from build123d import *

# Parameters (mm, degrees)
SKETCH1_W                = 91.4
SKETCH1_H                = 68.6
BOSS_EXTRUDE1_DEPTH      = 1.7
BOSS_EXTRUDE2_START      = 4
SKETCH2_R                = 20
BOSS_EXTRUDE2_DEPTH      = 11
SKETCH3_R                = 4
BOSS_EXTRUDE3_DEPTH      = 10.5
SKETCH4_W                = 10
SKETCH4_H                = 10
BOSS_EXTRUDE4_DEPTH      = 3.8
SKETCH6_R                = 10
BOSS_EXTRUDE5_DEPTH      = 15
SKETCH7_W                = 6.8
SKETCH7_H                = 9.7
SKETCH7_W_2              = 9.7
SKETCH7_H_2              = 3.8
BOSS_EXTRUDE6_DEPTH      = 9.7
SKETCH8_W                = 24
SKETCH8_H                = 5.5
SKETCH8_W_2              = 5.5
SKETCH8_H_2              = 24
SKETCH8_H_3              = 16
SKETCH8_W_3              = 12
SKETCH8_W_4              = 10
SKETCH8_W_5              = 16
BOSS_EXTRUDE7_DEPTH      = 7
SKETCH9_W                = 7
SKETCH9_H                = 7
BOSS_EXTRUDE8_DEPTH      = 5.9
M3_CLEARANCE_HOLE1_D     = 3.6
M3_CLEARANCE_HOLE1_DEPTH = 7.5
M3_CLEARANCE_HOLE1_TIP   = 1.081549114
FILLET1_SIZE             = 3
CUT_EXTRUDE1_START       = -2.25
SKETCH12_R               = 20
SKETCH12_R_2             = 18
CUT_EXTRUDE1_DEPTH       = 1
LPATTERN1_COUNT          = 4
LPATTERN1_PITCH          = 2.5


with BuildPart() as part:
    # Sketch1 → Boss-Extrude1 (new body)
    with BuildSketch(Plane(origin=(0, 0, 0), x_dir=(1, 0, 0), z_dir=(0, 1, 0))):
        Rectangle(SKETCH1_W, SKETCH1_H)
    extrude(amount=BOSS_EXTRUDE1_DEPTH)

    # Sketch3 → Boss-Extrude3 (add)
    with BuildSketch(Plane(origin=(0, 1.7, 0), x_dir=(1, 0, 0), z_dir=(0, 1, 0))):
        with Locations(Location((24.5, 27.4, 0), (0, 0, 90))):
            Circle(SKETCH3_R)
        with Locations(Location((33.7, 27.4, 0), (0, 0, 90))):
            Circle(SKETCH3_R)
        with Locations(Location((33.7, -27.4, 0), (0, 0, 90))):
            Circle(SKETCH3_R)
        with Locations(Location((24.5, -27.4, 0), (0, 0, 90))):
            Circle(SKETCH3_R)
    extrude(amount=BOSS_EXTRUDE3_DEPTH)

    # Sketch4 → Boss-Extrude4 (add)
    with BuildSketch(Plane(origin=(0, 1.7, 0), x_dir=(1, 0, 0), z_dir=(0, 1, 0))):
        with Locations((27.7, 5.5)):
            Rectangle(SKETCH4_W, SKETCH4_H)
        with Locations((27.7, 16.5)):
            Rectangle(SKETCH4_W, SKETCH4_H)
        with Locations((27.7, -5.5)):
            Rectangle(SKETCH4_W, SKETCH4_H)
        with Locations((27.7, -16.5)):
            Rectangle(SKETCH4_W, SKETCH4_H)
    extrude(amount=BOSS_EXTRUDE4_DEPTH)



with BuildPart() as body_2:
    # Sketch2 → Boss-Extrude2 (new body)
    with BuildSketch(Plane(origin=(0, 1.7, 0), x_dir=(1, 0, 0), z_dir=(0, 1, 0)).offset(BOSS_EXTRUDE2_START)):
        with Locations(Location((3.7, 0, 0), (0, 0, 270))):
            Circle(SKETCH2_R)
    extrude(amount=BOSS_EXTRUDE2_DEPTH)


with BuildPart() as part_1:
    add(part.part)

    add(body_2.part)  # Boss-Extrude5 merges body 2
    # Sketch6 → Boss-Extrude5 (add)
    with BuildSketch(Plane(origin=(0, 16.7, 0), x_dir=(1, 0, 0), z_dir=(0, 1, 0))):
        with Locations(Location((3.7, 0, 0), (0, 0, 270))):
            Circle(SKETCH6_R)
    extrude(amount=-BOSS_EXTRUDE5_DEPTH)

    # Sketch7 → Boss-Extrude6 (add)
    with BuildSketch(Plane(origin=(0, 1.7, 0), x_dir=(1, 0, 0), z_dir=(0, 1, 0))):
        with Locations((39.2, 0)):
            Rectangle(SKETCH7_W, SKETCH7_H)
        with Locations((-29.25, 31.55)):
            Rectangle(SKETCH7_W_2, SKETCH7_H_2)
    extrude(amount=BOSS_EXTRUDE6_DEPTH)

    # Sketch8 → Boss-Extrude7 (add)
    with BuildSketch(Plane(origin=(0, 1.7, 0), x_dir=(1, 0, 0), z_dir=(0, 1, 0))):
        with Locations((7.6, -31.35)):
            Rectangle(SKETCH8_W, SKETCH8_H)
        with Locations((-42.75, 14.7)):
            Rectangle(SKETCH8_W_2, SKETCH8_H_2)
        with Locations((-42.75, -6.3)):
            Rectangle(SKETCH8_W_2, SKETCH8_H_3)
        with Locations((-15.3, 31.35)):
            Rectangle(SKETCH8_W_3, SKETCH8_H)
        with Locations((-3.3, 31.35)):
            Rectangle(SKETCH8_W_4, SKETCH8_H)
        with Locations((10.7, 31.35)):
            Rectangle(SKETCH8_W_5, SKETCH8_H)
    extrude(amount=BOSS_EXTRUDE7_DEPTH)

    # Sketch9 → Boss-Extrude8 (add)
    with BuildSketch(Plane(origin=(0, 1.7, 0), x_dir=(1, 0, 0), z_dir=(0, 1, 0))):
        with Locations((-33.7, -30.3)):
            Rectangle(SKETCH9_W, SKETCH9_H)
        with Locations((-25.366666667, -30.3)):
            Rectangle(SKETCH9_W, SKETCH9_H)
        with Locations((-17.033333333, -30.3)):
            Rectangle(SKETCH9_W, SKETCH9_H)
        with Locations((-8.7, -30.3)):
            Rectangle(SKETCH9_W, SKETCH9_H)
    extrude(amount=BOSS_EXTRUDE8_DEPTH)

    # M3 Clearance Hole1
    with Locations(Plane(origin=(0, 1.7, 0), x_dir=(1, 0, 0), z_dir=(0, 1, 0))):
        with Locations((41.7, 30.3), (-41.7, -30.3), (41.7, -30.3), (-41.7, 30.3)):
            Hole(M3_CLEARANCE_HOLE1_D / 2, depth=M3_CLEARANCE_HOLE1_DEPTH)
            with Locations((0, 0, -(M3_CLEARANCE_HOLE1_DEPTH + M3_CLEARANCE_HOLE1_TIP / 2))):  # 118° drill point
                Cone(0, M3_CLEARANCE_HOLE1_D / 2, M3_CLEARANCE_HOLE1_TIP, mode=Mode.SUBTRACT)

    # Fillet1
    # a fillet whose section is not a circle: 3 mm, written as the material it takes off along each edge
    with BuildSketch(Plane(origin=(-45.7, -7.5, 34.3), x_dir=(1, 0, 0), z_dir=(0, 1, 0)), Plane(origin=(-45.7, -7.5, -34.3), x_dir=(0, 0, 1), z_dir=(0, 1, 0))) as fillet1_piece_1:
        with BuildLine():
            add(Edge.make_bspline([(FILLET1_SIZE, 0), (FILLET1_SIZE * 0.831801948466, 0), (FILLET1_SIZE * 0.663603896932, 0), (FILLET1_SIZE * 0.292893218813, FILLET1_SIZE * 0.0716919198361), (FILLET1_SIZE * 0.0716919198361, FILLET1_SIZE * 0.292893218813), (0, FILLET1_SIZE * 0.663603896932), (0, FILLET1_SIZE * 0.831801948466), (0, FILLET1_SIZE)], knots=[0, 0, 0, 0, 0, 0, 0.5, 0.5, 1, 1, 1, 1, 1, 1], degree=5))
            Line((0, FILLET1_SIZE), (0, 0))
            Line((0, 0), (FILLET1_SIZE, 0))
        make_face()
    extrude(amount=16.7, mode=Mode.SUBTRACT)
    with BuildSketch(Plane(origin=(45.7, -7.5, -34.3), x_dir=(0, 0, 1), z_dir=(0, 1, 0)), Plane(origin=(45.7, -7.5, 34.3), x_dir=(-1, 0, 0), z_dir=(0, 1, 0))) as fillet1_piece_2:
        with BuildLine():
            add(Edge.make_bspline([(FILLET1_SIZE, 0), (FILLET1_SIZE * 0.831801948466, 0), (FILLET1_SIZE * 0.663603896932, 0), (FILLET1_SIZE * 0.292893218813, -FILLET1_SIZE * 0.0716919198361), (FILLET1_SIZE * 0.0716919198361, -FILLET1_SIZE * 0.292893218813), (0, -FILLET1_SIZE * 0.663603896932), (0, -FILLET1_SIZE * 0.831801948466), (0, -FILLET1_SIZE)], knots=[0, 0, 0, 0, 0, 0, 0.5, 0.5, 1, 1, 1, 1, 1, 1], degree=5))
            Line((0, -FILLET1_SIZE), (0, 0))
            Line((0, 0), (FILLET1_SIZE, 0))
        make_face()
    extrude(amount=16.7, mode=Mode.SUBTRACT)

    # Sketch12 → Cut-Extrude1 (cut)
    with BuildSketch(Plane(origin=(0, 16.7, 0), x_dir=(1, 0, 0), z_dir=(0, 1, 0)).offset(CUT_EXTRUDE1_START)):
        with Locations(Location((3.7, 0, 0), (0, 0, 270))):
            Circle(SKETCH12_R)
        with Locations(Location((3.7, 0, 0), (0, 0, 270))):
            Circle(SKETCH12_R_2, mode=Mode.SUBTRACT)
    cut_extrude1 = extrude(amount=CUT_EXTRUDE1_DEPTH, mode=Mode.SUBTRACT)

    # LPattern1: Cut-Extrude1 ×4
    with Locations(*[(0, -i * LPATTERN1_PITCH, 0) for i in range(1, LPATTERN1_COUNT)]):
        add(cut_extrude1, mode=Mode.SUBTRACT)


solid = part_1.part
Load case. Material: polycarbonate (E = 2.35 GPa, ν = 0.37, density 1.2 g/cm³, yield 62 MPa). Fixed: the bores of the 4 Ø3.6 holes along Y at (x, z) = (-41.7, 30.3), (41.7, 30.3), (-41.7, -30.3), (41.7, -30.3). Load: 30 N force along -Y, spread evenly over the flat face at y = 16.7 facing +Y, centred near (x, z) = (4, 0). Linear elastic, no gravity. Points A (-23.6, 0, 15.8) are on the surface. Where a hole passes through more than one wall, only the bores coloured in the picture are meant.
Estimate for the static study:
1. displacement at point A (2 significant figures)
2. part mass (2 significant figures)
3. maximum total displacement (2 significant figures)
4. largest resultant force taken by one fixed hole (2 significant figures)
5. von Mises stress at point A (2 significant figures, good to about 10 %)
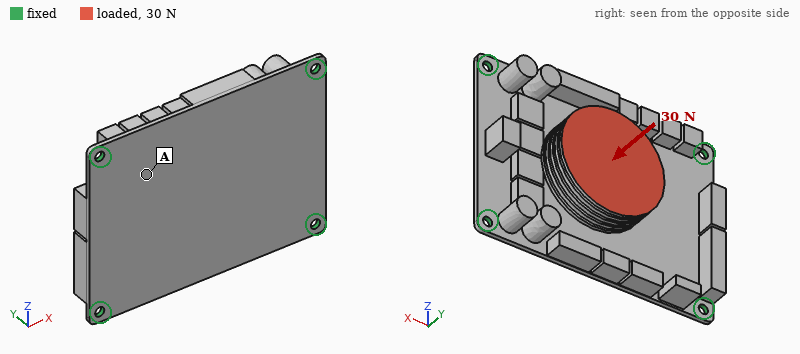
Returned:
0.55 mm
41 g
1.1 mm
9.8 N
1.5 MPa
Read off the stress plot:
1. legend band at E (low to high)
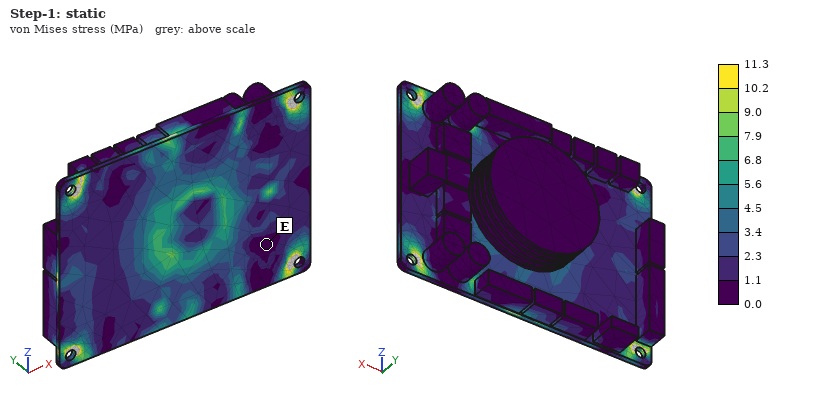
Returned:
0.0 to 1.1 MPa
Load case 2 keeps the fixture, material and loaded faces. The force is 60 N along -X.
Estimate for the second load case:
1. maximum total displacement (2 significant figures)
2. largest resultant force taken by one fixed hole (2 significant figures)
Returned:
1.4 mm
20 N
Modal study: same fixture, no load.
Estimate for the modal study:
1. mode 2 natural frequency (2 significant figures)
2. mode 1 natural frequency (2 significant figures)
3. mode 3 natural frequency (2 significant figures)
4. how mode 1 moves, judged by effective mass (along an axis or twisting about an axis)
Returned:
320 Hz
180 Hz
360 Hz
along Y
